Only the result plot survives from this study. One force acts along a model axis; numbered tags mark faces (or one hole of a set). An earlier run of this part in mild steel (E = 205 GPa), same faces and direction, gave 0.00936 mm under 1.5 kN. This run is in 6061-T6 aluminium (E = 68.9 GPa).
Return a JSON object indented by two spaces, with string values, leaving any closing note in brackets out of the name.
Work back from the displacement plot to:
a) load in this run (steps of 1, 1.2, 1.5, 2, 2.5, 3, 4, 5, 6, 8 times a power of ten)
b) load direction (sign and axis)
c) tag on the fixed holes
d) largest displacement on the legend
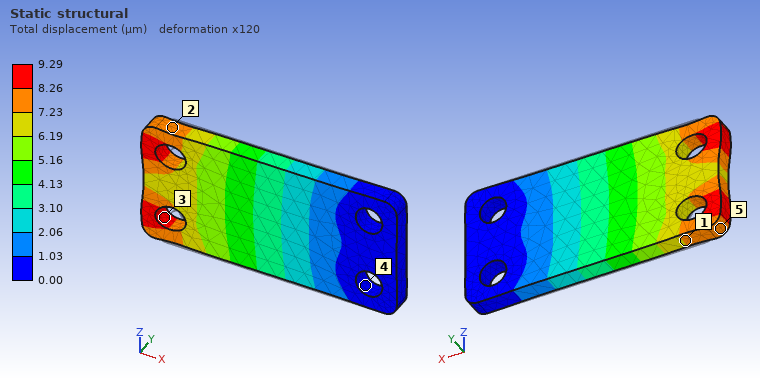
{
  "load in this run": "500 N",
  "load direction": "-X",
  "tag on the fixed holes": "4",
  "largest displacement on the legend": "9.29 µm"
}
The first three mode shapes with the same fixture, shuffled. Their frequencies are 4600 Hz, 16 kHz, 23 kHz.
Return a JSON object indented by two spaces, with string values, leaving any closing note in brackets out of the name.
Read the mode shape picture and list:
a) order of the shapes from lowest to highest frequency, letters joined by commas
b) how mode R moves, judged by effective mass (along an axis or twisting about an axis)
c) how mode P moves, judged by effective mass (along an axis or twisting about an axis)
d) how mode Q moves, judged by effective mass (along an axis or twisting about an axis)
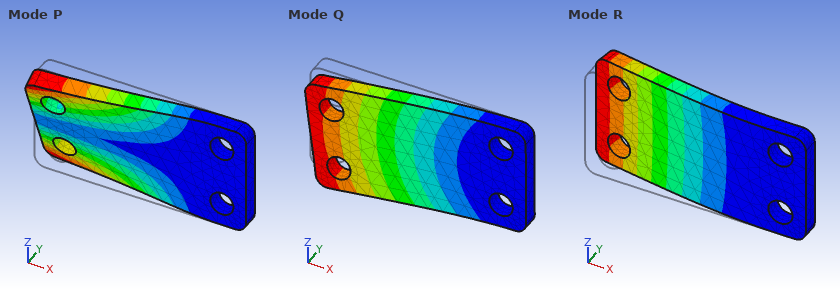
{
  "order of the shapes from lowest to highest frequency, letters joined by commas": "R, P, Q",
  "how mode R moves, judged by effective mass": "along Y",
  "how mode P moves, judged by effective mass": "twisting about X",
  "how mode Q moves, judged by effective mass": "along Z"
}
